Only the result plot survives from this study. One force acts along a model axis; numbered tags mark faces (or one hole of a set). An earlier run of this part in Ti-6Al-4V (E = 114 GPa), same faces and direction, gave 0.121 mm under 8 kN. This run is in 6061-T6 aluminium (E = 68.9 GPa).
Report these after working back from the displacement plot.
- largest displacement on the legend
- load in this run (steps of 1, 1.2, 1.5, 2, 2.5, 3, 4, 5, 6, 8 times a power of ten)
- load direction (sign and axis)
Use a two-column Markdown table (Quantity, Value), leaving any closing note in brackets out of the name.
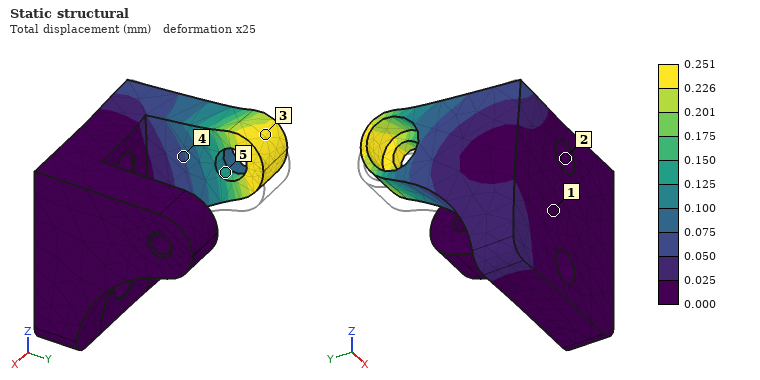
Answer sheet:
| Quantity | Value |
|---|---|
| largest displacement on the legend | 0.251 mm |
| load in this run | 10 kN |
| load direction | +Z |
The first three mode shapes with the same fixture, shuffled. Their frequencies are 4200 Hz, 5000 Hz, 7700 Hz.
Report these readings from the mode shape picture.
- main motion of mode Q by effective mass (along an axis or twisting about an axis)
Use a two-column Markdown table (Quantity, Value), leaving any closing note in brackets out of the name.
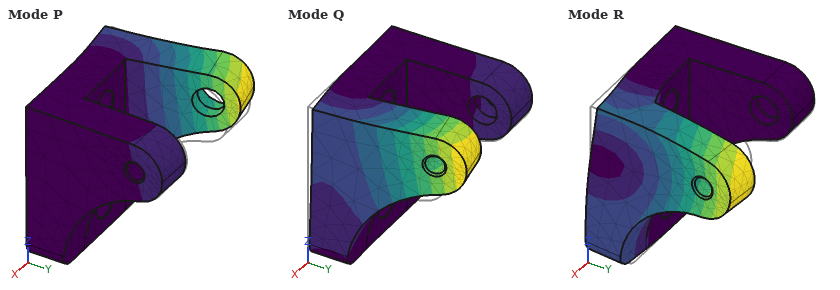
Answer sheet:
| Quantity | Value |
|---|---|
| main motion of mode Q by effective mass | along X |
